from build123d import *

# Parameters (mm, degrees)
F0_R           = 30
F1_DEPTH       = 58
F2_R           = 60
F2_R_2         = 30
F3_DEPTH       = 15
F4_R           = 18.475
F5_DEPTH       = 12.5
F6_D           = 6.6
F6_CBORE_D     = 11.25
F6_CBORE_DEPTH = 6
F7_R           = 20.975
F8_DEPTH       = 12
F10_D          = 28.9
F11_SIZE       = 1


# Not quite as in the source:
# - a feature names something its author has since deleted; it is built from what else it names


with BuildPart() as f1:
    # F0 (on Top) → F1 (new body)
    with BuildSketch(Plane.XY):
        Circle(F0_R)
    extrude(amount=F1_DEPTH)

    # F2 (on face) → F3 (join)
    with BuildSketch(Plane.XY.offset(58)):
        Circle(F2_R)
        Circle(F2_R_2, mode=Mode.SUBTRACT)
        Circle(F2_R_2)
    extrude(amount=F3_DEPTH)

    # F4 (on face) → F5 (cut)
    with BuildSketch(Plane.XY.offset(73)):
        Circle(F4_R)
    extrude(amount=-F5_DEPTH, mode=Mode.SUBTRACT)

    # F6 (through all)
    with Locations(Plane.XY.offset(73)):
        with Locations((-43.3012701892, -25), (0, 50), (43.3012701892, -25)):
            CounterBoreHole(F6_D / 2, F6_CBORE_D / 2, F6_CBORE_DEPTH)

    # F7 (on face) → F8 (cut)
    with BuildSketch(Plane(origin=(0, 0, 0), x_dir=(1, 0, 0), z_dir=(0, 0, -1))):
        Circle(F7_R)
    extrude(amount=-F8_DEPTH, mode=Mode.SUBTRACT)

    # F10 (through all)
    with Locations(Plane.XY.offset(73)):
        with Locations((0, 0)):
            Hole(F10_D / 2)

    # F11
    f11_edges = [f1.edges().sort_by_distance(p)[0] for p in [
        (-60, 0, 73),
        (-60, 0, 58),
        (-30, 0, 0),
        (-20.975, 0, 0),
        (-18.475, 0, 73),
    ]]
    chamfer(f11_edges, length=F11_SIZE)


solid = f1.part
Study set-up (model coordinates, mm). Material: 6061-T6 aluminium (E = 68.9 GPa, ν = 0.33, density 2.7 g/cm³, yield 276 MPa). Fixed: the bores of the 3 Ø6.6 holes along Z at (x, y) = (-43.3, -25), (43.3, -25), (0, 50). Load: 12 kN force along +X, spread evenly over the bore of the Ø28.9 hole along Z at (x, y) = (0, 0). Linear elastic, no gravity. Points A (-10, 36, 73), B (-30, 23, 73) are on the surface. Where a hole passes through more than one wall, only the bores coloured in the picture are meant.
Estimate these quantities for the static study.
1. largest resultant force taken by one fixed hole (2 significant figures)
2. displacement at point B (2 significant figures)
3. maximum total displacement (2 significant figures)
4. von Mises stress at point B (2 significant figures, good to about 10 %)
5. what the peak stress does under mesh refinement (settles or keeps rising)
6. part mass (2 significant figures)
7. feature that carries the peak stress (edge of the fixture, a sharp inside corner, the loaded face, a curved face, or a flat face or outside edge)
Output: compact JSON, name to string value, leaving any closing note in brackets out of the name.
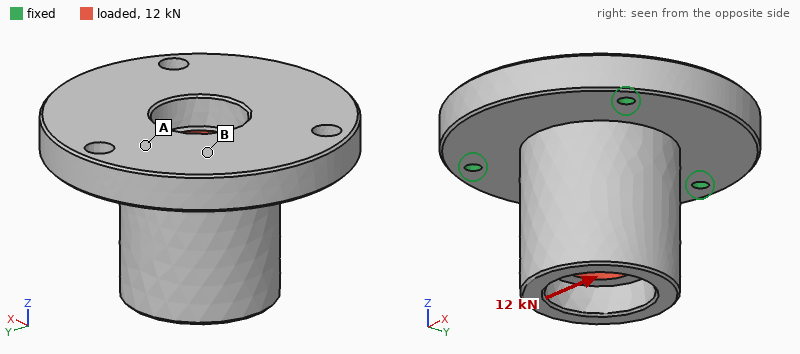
{"largest resultant force taken by one fixed hole": "5.3 kN", "displacement at point B": "22 µm", "maximum total displacement": "67 µm", "von Mises stress at point B": "14 MPa", "what the peak stress does under mesh refinement": "keeps rising", "part mass": "730 g", "feature that carries the peak stress": "edge of the fixture"}
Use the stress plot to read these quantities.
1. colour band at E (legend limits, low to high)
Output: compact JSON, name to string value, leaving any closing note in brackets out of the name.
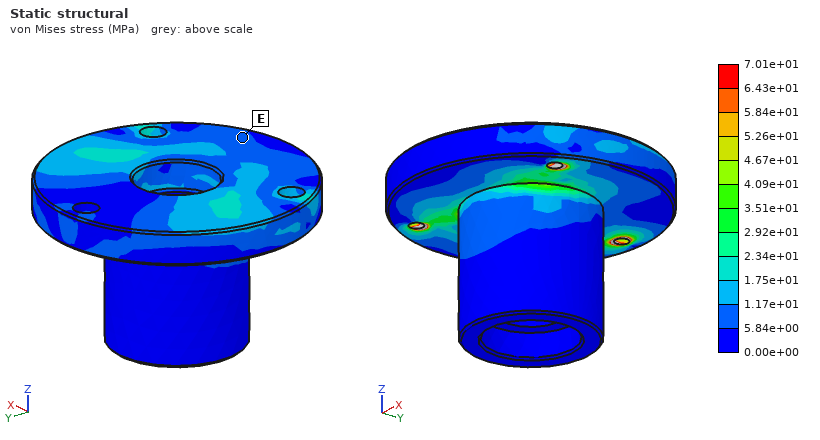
{"colour band at E": "5.84e+00 to 1.17e+01 MPa"}
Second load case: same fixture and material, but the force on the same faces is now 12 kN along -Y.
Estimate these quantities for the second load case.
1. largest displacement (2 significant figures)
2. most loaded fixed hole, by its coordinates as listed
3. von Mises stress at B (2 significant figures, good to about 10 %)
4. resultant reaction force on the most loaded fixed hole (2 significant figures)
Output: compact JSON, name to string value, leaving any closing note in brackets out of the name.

{"largest displacement": "68 µm", "most loaded fixed hole, by its coordinates as listed": "(0, 50)", "von Mises stress at B": "14 MPa", "resultant reaction force on the most loaded fixed hole": "5.6 kN"}
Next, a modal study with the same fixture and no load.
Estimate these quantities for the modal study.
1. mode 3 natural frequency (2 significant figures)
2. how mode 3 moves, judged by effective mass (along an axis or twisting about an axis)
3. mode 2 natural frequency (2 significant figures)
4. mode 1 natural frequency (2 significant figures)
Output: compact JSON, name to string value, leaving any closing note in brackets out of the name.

{"mode 3 natural frequency": "4500 Hz", "how mode 3 moves, judged by effective mass": "along Z", "mode 2 natural frequency": "3600 Hz", "mode 1 natural frequency": "3600 Hz"}
